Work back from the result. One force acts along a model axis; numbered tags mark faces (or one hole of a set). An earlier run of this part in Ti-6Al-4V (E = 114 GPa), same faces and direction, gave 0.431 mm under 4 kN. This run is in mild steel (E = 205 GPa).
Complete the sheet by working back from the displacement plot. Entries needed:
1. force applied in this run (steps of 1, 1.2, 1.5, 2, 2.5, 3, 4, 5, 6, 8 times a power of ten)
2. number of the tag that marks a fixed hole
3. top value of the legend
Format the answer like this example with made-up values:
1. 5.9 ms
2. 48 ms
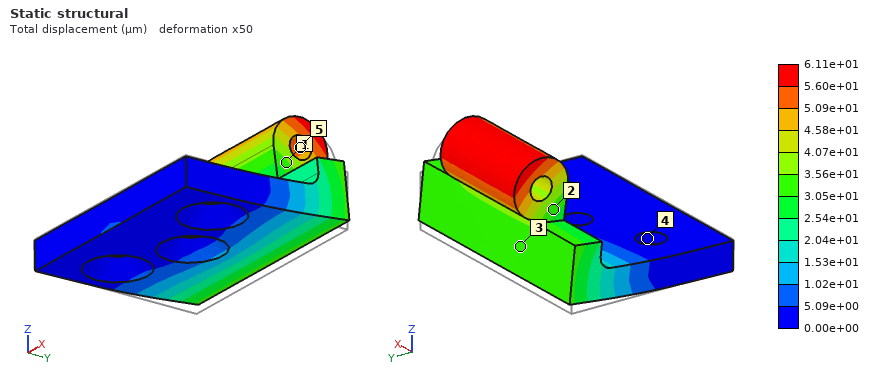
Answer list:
1. 1 kN
2. 4
3. 6.11e+01 µm
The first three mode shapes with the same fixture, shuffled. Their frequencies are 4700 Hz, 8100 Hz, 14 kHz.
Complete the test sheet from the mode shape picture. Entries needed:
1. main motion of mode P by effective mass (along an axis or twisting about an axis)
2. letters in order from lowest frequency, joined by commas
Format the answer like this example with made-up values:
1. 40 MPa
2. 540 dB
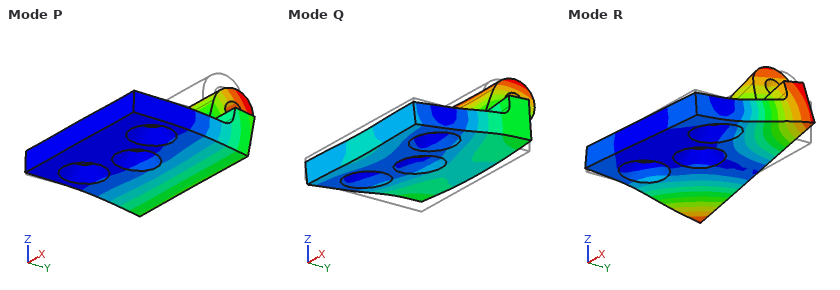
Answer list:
1. along Z
2. P, R, Q
